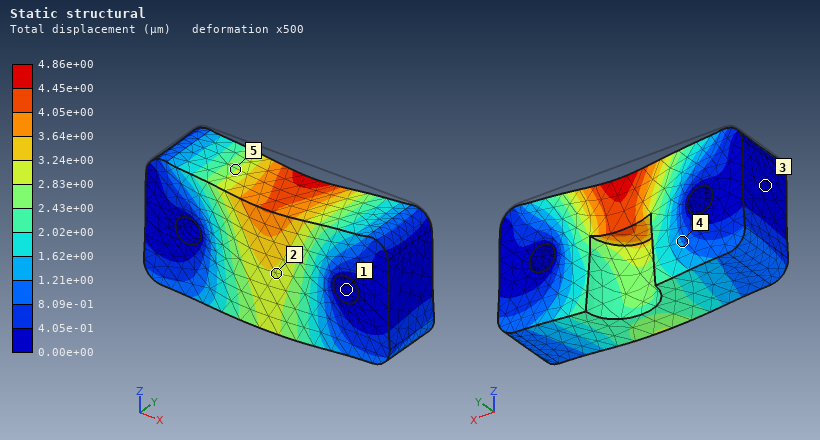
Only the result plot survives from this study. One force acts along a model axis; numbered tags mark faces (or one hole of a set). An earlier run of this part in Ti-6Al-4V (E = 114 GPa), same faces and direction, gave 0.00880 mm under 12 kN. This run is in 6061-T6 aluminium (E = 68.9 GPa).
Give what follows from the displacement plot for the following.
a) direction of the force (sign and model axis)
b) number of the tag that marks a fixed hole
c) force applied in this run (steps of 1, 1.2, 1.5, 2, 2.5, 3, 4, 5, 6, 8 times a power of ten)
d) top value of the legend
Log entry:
-Z
1
4 kN
4.86e+00 µm
